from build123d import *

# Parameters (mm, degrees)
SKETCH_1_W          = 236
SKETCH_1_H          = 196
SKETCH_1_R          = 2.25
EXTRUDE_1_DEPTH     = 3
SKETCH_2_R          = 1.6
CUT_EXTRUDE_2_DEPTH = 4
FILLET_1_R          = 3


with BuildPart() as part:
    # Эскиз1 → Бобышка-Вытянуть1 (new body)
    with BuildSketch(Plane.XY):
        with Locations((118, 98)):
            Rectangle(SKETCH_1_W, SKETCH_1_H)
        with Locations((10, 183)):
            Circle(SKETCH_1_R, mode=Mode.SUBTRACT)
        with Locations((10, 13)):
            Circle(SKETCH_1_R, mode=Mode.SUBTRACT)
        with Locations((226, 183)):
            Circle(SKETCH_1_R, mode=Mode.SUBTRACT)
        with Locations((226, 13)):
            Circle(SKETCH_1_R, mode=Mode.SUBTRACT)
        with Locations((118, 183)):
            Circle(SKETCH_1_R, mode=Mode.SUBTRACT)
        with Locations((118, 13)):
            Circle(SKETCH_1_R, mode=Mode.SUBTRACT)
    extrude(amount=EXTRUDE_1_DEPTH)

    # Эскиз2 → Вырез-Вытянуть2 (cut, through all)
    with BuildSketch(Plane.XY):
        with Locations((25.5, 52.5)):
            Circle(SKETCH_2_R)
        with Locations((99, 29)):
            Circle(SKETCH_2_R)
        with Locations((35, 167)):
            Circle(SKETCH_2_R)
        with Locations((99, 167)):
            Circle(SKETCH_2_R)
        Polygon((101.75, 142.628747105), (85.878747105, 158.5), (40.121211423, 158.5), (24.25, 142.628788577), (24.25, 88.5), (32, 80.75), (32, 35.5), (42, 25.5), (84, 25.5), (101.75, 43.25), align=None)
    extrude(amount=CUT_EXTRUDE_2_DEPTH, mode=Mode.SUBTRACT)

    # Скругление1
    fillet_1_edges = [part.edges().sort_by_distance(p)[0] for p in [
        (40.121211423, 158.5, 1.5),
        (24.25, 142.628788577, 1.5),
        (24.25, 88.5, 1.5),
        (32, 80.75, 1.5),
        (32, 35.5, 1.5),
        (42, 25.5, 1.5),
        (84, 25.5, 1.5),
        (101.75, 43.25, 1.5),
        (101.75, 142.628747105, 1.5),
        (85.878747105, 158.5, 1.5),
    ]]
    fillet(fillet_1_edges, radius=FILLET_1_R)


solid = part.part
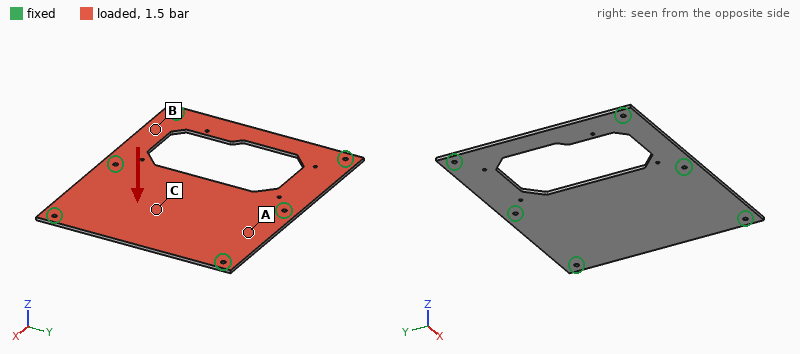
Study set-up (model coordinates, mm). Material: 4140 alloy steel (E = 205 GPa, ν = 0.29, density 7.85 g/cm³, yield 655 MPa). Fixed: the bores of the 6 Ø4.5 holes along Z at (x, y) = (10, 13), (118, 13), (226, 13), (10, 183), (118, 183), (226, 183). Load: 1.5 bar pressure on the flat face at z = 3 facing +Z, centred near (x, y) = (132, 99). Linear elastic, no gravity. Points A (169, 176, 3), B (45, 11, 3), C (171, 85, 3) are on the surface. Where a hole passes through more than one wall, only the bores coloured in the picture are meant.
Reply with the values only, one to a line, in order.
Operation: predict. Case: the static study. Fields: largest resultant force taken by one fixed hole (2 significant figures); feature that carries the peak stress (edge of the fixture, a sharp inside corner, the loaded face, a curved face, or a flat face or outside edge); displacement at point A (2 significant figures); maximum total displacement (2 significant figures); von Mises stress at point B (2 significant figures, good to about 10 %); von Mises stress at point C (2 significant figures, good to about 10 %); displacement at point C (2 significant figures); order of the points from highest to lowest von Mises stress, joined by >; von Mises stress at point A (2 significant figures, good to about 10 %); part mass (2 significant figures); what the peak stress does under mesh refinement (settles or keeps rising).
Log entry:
1.3 kN
edge of the fixture
0.27 mm
1.1 mm
36 MPa
110 MPa
1.0 mm
C > A > B
79 MPa
870 g
keeps rising
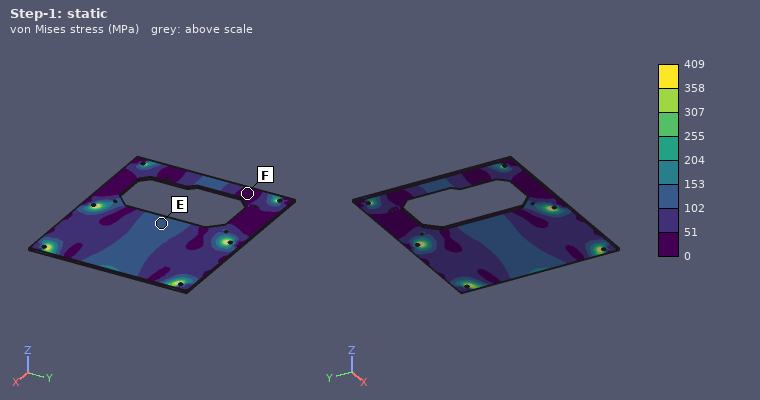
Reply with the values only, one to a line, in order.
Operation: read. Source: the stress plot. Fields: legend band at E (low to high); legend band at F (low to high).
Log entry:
102 to 153 MPa
0 to 51 MPa
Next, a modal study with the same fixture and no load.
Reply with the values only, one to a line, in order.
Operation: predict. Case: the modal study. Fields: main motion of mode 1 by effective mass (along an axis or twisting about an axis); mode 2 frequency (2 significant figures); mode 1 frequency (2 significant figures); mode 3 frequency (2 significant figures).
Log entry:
along Z
580 Hz
450 Hz
720 Hz
